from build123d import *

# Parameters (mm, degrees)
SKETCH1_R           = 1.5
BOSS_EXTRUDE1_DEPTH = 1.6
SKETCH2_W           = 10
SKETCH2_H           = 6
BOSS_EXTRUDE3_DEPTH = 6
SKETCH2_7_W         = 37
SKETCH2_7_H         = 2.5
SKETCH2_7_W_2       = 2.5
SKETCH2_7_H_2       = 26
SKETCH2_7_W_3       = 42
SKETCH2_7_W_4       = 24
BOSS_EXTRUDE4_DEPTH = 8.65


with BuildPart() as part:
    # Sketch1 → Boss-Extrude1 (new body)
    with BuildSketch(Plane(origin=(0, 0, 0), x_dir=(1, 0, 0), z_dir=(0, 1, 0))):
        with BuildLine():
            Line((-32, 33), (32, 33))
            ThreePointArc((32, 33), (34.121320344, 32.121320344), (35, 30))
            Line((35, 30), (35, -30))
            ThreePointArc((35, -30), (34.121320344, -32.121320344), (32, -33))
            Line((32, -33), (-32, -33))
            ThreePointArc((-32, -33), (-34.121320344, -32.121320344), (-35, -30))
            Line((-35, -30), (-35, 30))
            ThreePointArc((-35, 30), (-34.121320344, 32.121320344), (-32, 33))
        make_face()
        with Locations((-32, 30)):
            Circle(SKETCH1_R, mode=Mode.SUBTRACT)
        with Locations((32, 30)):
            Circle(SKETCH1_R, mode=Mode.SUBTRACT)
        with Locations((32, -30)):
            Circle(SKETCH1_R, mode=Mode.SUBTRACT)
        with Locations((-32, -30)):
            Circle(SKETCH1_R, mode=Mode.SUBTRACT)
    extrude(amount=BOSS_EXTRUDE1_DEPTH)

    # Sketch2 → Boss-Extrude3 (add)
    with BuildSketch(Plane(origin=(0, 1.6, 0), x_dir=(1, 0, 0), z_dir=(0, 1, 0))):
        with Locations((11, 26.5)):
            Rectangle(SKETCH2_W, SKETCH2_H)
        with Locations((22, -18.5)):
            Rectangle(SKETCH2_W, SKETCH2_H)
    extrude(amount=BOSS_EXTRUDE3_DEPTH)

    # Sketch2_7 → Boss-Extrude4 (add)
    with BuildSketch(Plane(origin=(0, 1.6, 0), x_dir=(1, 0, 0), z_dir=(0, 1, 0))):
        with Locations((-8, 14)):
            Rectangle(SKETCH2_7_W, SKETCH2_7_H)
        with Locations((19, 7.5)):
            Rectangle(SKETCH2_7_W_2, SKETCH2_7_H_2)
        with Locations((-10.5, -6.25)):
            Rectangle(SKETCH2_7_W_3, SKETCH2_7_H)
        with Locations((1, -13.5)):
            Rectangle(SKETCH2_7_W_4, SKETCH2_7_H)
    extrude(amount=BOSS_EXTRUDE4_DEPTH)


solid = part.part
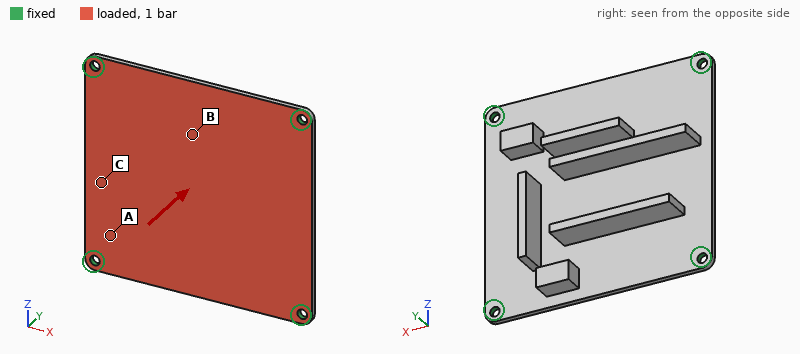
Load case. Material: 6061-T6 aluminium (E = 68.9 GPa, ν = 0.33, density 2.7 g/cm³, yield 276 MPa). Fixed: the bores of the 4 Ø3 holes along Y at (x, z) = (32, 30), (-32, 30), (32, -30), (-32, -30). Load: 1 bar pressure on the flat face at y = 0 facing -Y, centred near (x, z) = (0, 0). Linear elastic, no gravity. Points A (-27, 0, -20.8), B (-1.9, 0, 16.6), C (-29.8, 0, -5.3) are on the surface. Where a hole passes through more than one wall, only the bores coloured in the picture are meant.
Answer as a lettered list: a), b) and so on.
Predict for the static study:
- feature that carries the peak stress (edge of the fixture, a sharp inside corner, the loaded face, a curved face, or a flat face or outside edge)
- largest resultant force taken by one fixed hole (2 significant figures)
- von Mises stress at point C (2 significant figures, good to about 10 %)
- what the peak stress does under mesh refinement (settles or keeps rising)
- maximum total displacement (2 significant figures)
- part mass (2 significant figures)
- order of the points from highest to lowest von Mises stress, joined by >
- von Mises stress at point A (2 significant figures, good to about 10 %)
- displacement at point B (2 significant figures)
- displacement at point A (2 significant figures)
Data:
a) edge of the fixture
b) 120 N
c) 41 MPa
d) keeps rising
e) 0.28 mm
f) 29 g
g) C > A > B
h) 23 MPa
i) 0.23 mm
j) 0.093 mm
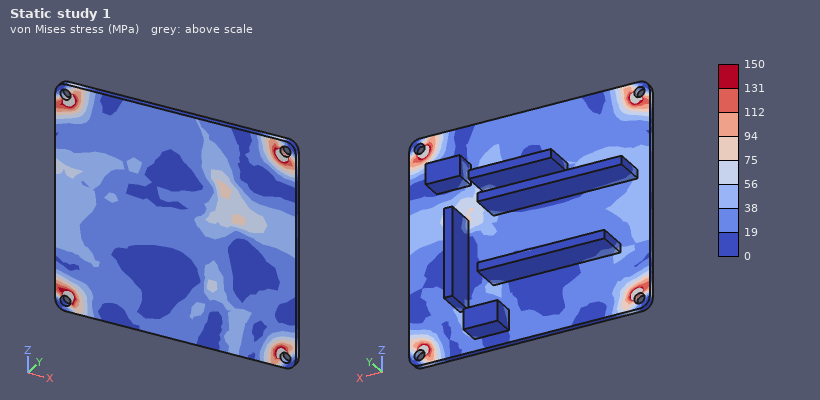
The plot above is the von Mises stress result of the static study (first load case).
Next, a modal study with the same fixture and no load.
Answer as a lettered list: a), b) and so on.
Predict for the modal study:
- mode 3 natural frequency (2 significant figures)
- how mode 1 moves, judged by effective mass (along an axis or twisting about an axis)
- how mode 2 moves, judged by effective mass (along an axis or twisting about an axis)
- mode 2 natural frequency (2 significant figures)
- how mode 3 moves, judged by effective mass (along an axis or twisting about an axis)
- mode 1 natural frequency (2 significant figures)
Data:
a) 2400 Hz
b) along Y
c) twisting about Z
d) 2300 Hz
e) twisting about X
f) 1300 Hz
